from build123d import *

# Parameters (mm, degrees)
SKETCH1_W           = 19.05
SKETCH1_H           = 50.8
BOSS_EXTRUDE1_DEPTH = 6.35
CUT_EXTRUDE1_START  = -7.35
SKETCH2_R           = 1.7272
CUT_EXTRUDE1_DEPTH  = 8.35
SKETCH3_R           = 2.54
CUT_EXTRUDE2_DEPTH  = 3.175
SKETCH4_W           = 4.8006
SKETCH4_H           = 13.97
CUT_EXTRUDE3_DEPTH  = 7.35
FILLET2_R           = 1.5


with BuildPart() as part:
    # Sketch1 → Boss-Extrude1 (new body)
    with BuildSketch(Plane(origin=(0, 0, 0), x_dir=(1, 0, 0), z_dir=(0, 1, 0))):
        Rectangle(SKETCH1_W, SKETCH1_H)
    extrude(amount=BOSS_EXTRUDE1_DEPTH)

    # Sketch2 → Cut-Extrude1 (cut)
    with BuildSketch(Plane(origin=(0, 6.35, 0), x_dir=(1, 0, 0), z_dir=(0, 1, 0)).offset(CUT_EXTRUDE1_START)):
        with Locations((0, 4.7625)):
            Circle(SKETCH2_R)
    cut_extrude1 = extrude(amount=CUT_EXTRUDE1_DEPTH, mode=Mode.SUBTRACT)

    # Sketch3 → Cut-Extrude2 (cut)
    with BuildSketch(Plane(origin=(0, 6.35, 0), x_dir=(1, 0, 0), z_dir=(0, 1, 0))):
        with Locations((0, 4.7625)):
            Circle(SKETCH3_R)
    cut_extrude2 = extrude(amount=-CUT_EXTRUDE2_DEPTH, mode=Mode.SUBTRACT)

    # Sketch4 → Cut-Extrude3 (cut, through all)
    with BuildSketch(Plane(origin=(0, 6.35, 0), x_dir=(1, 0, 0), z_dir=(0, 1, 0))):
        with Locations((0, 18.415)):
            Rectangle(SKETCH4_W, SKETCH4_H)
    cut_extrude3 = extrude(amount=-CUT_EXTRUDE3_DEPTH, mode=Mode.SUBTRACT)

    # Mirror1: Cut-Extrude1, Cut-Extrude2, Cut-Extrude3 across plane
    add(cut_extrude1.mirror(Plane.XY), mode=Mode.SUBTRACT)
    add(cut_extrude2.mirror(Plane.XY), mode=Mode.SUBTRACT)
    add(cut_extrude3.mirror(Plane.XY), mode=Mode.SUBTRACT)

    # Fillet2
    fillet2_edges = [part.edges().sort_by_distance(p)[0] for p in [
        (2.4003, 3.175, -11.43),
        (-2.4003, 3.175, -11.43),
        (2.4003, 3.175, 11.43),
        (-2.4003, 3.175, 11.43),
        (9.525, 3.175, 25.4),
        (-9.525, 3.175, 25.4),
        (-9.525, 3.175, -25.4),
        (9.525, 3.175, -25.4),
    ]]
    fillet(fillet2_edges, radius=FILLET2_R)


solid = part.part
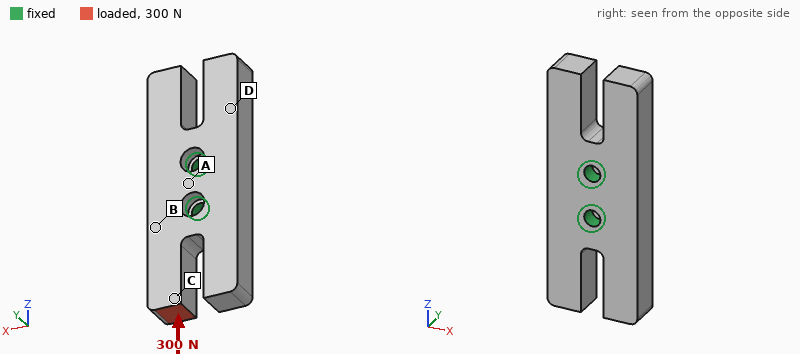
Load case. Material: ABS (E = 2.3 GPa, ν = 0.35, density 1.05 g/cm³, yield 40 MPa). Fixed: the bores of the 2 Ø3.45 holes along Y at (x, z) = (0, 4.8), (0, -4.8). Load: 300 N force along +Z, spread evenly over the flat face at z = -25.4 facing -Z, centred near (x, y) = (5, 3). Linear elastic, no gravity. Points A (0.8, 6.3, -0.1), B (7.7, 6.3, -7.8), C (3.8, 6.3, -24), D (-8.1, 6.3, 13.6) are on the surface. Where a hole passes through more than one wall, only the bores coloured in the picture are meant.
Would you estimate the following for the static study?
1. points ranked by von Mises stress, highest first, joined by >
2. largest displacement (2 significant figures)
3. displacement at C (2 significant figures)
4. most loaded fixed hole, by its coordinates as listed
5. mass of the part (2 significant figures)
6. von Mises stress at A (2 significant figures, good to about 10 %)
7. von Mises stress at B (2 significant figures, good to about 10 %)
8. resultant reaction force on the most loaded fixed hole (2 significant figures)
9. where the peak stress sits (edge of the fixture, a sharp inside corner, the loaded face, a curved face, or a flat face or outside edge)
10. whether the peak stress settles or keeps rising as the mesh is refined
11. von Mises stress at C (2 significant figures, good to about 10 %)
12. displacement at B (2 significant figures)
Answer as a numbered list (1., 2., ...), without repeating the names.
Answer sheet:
1. C > B > A > D
2. 0.11 mm
3. 0.10 mm
4. (0, -4.8)
5. 5.4 g
6. 2.8 MPa
7. 6.4 MPa
8. 230 N
9. edge of the fixture
10. keeps rising
11. 8.7 MPa
12. 0.049 mm
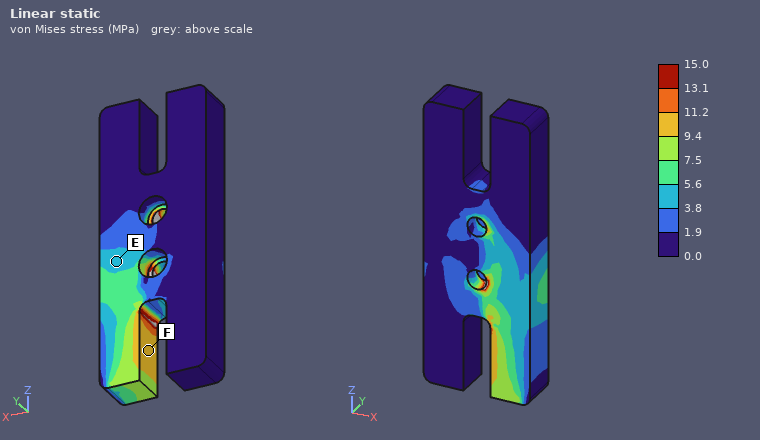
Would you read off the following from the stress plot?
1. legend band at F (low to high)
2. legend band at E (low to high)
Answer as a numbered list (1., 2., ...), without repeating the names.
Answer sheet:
1. 9.4 to 11.2 MPa
2. 3.8 to 5.6 MPa
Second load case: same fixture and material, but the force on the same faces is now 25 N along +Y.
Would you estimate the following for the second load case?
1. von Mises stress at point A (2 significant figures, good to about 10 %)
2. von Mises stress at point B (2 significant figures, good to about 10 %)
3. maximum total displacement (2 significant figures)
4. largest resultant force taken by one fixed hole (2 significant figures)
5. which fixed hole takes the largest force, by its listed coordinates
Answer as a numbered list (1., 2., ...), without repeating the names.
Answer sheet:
1. 1.9 MPa
2. 6.3 MPa
3. 0.26 mm
4. 63 N
5. (0, -4.8)
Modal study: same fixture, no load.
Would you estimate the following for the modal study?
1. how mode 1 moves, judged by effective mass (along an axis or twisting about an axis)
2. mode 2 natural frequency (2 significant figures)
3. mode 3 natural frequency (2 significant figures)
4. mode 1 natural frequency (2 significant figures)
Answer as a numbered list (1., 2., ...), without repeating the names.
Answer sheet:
1. twisting about X
2. 3000 Hz
3. 3000 Hz
4. 2700 Hz
